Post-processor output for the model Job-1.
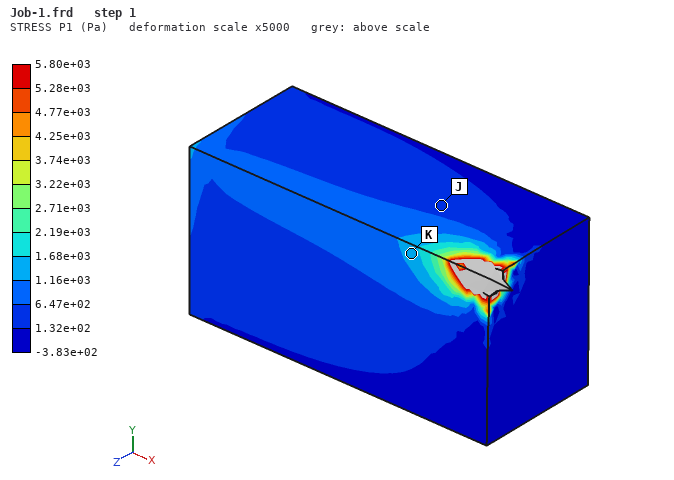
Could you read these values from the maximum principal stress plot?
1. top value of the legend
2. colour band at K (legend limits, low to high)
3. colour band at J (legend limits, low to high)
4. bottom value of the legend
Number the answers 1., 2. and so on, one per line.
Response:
1. 5.80e+03 Pa
2. 1.16e+03 to 1.68e+03 Pa
3. 1.32e+02 to 6.47e+02 Pa
4. -3.83e+02 Pa
